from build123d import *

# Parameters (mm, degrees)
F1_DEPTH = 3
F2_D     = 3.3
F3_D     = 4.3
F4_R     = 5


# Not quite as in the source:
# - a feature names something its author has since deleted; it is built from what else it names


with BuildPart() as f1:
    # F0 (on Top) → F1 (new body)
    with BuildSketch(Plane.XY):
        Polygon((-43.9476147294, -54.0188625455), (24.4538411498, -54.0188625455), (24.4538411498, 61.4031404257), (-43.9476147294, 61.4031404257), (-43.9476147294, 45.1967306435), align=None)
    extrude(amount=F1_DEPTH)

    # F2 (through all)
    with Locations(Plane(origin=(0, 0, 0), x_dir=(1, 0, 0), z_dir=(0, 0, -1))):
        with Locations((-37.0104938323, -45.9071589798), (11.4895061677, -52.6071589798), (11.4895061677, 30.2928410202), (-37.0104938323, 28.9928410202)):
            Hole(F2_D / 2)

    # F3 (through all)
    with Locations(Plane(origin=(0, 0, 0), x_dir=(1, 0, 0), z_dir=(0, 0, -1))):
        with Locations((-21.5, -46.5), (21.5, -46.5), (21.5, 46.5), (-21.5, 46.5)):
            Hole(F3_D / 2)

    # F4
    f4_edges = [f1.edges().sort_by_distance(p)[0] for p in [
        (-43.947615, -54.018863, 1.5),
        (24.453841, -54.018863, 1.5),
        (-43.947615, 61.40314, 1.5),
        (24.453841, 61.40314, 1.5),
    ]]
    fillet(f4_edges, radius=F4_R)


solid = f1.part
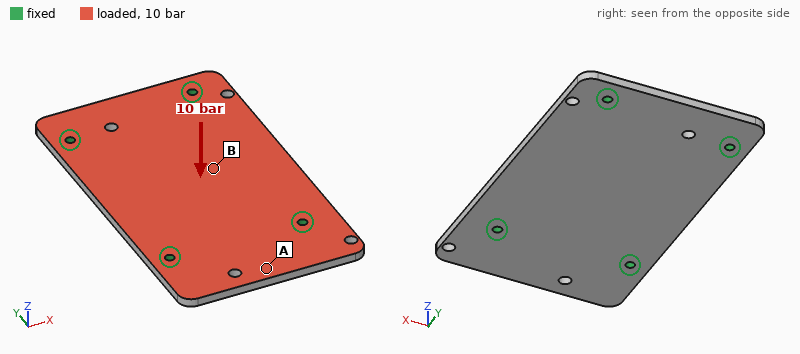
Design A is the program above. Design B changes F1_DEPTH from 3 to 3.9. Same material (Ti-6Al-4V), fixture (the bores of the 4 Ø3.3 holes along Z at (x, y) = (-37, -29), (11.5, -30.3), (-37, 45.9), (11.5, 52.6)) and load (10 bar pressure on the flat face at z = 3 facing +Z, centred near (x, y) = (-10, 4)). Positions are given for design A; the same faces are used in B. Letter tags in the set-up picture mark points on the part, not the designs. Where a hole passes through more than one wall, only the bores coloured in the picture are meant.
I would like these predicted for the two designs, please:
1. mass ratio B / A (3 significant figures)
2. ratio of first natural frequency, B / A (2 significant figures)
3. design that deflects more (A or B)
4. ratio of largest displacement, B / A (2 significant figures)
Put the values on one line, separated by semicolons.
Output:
1.30; 1.3; A; 0.47
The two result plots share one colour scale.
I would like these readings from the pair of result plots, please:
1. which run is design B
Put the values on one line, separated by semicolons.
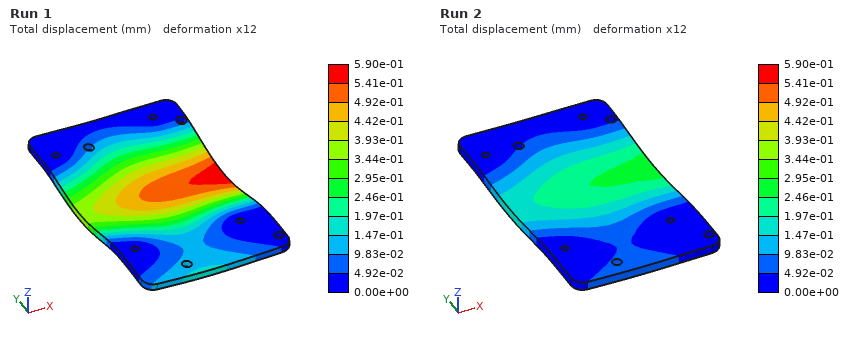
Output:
Run 2
